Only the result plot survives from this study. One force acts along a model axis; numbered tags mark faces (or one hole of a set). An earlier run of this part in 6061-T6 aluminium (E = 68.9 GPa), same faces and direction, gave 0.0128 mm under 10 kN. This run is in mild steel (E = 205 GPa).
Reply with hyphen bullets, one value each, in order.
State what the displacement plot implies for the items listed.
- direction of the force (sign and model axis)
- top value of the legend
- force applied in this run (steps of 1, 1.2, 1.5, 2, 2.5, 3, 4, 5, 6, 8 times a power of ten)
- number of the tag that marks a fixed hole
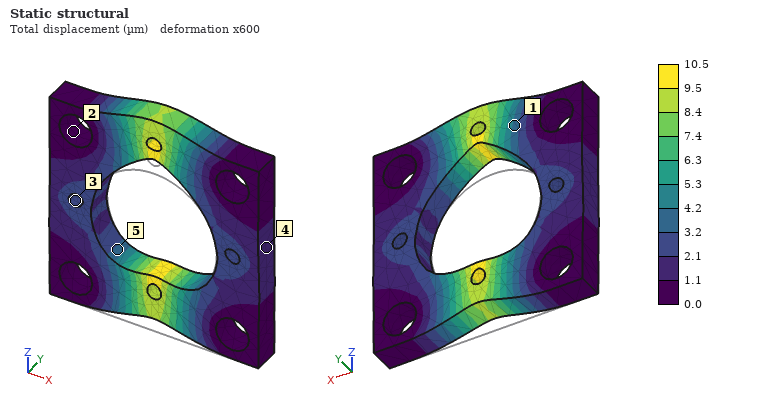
- +Z
- 10.5 µm
- 25 kN
- 2
